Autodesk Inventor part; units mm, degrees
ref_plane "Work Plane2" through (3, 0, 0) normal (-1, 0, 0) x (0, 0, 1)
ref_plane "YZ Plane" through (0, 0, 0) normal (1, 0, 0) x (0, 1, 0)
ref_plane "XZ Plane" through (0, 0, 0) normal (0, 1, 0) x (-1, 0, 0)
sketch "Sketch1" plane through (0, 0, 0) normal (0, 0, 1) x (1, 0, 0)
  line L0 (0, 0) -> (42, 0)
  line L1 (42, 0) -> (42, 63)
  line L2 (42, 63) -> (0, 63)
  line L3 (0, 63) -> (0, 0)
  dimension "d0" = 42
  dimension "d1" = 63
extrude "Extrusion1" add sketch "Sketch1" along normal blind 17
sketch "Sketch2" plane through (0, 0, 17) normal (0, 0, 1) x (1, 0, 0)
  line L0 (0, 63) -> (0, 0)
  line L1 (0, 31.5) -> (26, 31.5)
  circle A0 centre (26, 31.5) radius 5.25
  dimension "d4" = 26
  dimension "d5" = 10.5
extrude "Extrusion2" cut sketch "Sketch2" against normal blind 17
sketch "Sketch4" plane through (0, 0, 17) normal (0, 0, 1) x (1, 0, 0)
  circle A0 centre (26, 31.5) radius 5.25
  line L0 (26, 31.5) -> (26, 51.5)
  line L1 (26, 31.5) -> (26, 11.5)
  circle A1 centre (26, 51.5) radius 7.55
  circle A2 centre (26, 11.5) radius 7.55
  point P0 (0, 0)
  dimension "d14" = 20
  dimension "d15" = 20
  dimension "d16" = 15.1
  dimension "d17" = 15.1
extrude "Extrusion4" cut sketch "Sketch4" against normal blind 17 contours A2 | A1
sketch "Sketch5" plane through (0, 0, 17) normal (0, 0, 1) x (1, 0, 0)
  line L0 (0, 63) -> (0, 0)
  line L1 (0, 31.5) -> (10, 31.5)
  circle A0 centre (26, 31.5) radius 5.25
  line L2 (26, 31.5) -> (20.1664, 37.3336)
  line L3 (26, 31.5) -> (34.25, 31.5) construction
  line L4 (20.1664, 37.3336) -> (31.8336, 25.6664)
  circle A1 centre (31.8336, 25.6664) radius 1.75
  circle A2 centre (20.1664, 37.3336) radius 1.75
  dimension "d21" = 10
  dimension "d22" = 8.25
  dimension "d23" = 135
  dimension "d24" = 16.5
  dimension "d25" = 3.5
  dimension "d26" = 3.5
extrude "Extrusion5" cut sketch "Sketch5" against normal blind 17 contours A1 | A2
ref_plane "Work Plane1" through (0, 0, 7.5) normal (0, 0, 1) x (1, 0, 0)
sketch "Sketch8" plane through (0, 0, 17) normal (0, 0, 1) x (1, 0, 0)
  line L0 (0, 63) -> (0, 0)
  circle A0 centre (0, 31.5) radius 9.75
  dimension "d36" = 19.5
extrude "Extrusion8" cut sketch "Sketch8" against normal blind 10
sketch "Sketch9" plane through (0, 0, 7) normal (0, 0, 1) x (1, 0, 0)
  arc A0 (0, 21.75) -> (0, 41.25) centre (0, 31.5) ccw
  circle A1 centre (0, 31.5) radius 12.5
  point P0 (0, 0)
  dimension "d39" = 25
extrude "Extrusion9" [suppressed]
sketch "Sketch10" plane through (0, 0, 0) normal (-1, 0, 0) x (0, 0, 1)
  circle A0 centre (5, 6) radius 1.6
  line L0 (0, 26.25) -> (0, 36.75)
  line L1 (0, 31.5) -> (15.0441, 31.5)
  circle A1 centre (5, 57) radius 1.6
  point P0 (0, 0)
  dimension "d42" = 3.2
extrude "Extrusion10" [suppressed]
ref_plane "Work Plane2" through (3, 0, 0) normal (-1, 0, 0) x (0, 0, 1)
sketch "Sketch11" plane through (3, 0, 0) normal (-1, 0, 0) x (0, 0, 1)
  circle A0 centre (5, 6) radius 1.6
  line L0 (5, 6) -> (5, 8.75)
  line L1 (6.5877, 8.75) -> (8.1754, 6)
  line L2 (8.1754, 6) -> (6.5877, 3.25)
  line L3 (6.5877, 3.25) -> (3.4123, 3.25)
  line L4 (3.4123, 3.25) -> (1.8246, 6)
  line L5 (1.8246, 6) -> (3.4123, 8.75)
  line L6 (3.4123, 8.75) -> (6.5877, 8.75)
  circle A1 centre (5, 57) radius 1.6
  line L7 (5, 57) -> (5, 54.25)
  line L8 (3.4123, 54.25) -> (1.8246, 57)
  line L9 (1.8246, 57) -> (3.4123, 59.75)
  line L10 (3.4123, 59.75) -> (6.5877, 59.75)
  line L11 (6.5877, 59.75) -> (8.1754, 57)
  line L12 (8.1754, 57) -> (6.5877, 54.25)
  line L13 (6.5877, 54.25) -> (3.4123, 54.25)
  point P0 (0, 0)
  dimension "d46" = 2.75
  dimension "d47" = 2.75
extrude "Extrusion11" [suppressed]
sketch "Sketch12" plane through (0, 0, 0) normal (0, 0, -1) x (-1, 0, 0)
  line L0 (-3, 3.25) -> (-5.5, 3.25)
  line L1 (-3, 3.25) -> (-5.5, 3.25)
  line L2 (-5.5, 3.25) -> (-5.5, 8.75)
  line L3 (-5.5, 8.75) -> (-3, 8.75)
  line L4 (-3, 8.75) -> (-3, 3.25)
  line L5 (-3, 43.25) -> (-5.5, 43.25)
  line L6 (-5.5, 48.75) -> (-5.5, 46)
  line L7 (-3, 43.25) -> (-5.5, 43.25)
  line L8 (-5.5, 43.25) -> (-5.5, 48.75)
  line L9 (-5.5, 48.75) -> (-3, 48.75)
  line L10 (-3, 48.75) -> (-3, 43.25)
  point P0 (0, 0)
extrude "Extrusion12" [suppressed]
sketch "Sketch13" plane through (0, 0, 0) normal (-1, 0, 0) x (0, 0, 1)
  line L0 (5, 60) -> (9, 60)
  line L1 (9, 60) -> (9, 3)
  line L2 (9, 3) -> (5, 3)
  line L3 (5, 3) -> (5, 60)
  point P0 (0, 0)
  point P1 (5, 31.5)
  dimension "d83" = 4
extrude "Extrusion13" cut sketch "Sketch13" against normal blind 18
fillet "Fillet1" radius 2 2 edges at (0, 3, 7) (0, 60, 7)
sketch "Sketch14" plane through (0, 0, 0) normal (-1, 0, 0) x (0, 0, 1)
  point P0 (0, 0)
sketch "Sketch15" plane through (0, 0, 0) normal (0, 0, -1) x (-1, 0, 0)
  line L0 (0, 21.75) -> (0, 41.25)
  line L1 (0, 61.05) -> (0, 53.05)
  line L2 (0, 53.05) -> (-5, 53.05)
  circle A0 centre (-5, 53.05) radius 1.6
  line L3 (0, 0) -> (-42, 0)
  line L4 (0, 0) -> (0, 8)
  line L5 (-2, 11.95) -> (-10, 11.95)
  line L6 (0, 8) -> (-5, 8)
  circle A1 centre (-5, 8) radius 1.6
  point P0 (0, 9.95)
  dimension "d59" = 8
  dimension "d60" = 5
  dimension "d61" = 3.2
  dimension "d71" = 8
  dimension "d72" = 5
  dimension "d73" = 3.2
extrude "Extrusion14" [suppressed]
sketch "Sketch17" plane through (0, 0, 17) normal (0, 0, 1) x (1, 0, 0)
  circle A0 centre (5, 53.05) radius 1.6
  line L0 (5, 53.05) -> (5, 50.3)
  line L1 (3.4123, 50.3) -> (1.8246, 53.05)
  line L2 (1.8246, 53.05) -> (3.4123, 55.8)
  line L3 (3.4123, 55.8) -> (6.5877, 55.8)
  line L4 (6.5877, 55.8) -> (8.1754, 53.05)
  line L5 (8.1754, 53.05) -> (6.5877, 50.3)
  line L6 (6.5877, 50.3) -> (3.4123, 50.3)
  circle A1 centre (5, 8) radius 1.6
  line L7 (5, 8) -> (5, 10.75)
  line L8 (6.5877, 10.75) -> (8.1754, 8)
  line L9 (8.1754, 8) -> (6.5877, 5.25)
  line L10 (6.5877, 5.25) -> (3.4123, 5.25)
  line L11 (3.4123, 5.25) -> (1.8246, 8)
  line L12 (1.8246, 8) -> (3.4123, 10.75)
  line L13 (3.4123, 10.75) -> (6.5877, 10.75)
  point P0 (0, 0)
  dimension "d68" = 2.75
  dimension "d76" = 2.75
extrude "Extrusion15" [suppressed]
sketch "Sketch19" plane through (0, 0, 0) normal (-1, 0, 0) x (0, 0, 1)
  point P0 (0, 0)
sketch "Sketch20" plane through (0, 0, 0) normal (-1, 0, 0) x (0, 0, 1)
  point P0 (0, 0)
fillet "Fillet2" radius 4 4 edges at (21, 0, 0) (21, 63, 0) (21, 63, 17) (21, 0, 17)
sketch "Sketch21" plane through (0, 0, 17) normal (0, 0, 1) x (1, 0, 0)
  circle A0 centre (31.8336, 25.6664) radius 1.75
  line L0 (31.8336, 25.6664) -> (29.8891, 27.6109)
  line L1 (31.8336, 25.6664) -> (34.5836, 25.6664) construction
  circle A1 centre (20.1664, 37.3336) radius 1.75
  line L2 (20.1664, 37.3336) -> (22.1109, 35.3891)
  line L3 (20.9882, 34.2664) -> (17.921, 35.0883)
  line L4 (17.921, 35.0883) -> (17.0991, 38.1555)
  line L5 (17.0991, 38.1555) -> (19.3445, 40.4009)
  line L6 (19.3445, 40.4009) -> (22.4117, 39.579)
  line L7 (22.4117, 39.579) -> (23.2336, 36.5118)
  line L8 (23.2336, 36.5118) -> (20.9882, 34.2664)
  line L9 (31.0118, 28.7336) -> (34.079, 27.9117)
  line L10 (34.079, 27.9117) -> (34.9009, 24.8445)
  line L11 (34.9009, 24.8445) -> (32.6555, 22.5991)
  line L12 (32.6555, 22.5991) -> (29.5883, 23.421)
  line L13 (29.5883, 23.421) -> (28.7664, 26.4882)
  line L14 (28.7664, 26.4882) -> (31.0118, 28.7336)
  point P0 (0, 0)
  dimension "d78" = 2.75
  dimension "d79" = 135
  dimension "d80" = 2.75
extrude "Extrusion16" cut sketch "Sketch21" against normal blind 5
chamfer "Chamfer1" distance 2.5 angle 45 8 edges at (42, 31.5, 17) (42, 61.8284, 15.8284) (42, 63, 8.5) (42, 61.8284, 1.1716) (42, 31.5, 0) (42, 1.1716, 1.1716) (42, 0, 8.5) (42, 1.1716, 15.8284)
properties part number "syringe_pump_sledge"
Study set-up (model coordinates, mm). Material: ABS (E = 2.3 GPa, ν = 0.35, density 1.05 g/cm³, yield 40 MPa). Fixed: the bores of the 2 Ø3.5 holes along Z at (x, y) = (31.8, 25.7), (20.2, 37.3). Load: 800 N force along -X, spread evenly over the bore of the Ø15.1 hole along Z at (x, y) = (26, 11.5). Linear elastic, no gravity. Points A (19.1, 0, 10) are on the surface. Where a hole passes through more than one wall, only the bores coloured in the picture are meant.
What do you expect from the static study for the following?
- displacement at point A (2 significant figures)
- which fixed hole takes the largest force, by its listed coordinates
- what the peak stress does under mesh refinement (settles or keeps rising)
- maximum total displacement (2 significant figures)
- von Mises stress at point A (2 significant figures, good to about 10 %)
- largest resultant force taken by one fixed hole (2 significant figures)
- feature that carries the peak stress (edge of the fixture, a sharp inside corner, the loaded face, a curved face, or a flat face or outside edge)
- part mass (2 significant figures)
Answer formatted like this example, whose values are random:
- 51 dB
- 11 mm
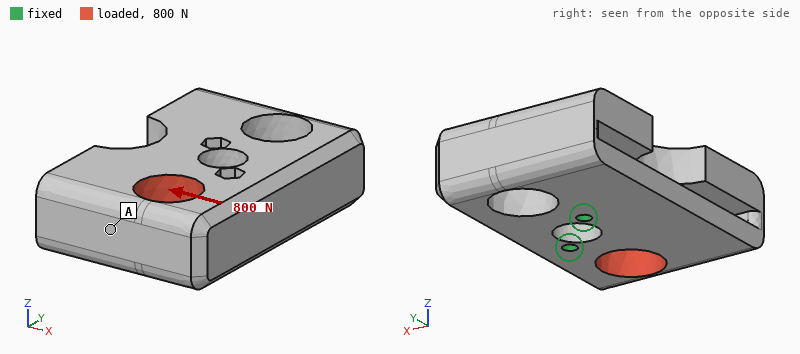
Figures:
- 0.19 mm
- (31.8, 25.7)
- keeps rising
- 0.24 mm
- 2.5 MPa
- 1.2 kN
- edge of the fixture
- 32 g
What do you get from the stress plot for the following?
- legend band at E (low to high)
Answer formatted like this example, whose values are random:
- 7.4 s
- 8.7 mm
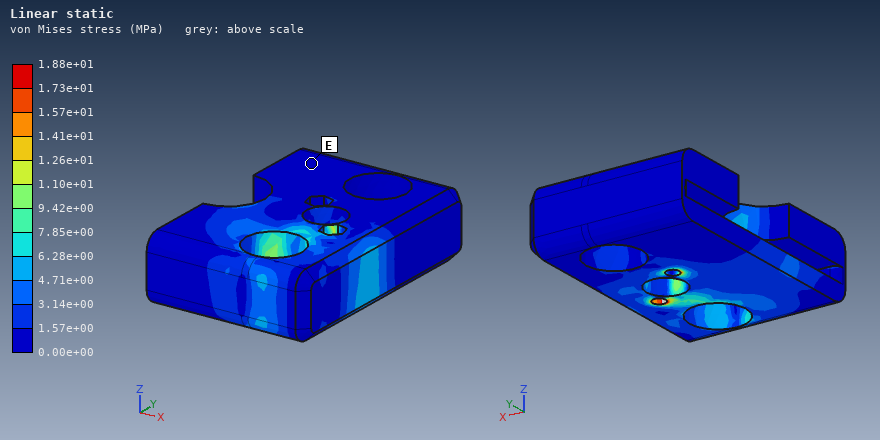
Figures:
- 0.00e+00 to 1.57e+00 MPa
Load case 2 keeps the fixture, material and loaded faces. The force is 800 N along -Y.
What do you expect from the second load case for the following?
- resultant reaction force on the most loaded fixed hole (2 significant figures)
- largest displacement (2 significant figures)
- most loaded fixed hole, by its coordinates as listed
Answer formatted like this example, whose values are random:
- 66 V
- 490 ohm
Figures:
- 430 N
- 70 µm
- (31.8, 25.7)
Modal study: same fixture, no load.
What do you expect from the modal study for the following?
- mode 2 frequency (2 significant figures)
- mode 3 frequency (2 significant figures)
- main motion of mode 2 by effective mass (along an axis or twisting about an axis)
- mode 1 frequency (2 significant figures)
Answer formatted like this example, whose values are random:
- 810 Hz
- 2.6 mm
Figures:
- 2300 Hz
- 2500 Hz
- along Z
- 1700 Hz
